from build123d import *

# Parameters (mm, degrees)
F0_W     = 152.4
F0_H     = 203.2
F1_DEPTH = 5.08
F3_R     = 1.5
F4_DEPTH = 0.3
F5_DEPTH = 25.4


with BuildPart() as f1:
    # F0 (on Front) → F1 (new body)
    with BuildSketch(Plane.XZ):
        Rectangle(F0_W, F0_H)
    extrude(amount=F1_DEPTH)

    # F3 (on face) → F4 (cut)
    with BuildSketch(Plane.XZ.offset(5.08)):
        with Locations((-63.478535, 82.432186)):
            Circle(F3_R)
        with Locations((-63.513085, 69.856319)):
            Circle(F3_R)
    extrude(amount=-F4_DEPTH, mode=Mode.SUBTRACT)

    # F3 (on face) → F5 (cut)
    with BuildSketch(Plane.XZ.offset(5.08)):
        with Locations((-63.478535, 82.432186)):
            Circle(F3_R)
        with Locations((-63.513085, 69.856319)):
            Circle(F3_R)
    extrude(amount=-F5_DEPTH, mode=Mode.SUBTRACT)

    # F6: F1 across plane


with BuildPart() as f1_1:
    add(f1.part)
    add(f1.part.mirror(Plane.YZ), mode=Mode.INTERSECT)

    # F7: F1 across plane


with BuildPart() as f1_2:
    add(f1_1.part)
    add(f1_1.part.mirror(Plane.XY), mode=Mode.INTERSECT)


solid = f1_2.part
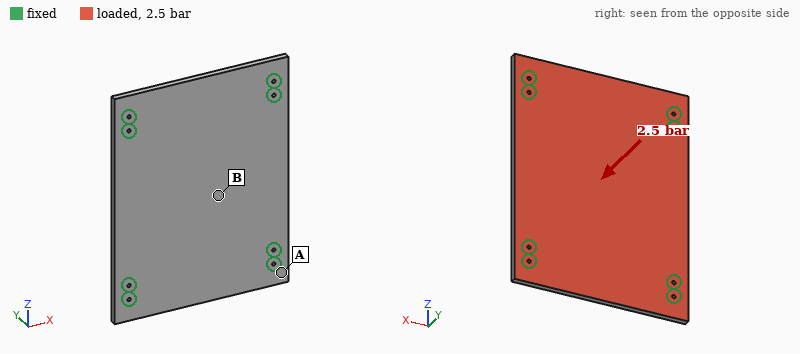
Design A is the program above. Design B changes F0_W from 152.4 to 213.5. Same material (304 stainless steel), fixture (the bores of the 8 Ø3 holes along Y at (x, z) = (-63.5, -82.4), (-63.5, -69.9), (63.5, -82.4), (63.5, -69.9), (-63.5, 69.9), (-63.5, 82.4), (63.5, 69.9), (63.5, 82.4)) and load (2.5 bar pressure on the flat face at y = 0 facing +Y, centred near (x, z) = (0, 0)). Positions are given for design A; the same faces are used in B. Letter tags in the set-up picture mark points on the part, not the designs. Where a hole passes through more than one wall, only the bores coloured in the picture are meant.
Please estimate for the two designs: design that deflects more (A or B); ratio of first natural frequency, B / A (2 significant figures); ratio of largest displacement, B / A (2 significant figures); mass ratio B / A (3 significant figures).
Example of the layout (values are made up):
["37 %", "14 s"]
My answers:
["A", "1.0", "0.88", "1.40"]
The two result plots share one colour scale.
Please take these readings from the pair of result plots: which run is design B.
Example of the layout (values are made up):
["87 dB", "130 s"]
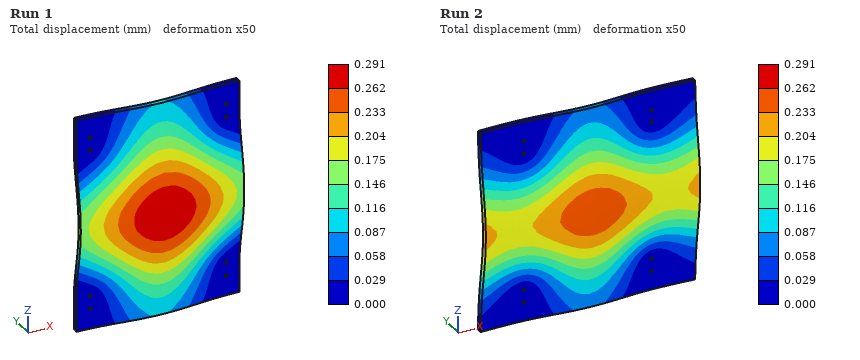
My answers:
["Run 2"]
